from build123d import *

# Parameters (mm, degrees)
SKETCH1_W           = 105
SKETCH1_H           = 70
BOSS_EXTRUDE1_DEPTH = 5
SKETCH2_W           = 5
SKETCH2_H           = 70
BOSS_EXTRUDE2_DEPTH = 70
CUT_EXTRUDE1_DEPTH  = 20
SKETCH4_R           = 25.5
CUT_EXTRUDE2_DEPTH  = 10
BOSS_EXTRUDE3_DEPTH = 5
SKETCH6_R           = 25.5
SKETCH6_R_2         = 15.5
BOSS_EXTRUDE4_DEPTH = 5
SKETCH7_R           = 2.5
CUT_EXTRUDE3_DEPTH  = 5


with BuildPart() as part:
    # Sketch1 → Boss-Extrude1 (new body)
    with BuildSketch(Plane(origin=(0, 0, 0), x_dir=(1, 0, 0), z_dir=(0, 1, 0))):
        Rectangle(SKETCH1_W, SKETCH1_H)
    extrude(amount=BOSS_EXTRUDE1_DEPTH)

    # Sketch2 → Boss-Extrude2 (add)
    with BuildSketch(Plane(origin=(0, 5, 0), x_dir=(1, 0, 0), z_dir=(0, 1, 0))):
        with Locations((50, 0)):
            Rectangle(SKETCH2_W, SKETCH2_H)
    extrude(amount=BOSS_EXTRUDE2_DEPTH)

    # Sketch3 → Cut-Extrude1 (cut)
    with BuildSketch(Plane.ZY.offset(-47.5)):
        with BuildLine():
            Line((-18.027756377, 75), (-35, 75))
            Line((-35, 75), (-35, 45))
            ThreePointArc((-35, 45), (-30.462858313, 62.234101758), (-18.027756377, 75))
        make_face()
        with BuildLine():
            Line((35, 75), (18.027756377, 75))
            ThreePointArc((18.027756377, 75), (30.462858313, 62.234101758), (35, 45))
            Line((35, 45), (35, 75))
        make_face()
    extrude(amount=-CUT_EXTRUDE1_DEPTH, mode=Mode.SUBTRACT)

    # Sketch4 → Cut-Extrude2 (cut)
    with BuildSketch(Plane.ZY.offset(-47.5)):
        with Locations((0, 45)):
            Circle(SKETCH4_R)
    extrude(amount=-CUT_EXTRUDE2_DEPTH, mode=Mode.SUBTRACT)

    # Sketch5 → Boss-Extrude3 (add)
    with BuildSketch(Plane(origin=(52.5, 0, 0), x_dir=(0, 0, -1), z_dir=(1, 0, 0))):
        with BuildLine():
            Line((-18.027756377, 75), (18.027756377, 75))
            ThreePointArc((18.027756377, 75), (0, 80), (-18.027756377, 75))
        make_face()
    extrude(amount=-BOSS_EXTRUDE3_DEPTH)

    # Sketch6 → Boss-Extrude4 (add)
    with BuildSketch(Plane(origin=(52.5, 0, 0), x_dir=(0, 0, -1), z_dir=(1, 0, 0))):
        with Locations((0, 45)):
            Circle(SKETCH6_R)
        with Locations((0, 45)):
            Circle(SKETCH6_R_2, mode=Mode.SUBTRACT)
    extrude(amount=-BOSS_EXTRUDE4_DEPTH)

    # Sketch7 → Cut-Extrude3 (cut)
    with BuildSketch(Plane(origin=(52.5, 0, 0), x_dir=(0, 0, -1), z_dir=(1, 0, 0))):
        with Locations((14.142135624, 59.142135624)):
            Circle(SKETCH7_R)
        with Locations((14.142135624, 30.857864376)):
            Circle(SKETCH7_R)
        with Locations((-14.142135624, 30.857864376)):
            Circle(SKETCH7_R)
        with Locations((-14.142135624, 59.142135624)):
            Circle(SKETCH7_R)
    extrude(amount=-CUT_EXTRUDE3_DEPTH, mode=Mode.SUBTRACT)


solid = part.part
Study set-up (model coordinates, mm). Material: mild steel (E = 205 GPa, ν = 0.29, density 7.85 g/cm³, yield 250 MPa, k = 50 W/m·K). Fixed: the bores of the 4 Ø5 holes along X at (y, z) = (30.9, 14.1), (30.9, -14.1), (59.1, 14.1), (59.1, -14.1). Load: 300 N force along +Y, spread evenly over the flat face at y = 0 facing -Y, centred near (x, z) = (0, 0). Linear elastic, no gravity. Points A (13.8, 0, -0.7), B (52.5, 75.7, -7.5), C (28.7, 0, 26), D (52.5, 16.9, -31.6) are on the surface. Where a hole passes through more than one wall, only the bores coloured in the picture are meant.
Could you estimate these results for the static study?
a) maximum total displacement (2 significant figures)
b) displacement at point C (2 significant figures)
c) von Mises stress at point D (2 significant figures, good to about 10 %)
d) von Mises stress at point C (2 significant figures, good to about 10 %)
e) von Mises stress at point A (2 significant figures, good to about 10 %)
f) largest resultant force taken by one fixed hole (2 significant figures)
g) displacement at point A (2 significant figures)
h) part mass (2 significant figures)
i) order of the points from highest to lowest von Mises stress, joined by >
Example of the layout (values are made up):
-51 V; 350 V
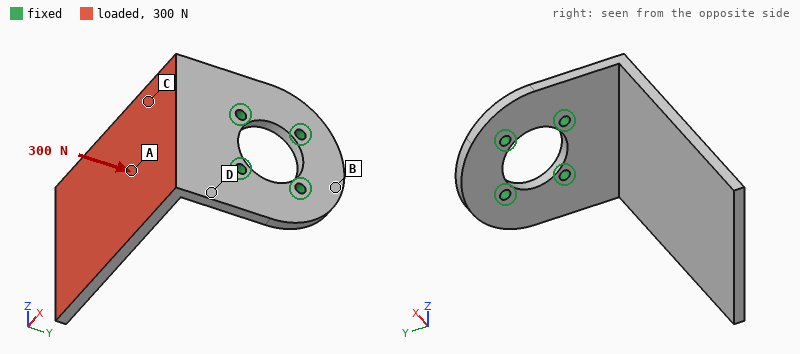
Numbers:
0.54 mm; 0.095 mm; 50 MPa; 31 MPa; 19 MPa; 170 N; 0.16 mm; 440 g; D > C > A > B
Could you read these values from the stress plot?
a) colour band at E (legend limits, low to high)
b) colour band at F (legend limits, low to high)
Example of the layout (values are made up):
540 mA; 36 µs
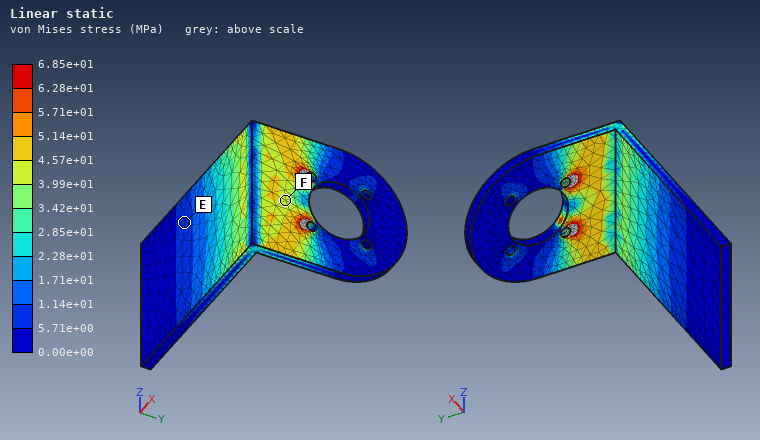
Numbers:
5.71e+00 to 1.14e+01 MPa; 3.99e+01 to 4.57e+01 MPa
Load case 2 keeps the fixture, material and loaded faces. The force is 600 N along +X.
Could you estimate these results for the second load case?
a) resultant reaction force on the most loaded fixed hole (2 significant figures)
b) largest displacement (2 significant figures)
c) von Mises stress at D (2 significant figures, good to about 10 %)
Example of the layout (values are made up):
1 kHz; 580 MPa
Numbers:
380 N; 0.25 mm; 33 MPa
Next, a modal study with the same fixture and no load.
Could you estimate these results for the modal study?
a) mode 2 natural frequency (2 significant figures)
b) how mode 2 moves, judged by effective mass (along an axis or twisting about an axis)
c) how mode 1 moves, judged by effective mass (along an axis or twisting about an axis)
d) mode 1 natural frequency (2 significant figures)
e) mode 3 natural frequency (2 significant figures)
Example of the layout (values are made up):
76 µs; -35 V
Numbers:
620 Hz; along Z; along Y; 270 Hz; 1300 Hz
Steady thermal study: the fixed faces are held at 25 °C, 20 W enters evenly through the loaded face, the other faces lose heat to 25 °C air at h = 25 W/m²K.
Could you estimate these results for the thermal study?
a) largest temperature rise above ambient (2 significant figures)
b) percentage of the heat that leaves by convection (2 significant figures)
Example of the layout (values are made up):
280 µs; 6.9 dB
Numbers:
48 K; 48 %
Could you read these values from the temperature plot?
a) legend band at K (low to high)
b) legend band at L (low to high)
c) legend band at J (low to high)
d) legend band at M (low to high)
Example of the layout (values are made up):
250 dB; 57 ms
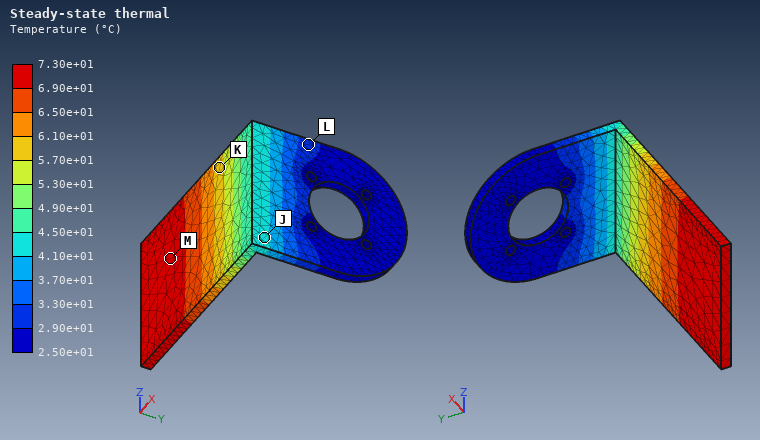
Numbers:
5.70e+01 to 6.10e+01 °C; 2.90e+01 to 3.30e+01 °C; 4.10e+01 to 4.50e+01 °C; 6.90e+01 to 7.30e+01 °C
